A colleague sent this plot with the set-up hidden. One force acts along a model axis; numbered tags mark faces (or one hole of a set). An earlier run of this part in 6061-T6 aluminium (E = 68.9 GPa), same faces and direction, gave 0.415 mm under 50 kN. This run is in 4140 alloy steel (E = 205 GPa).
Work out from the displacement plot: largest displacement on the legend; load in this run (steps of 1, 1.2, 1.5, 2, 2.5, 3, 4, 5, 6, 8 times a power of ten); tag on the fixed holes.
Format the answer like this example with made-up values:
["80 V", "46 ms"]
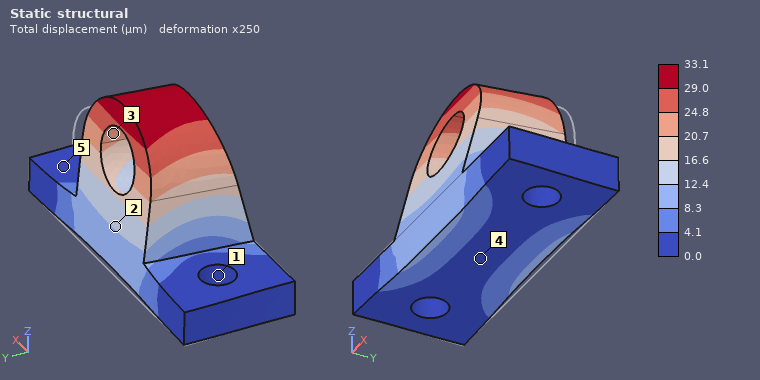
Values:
["33.1 µm", "12 kN", "1"]
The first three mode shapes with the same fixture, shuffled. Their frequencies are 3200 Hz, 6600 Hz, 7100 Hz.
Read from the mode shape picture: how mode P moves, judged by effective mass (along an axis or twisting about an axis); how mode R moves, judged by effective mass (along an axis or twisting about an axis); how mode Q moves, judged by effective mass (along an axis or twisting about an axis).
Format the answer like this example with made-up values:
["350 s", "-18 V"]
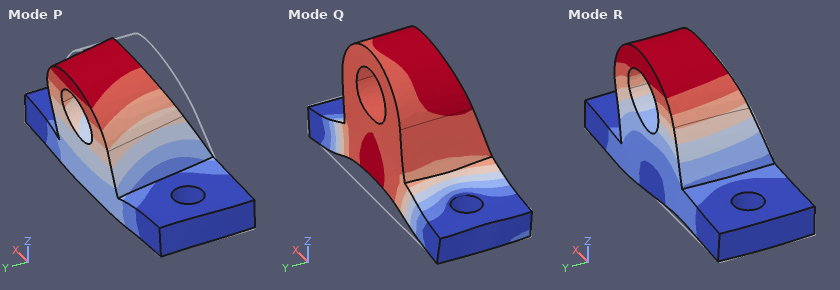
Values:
["along Y", "along X", "along Z"]
